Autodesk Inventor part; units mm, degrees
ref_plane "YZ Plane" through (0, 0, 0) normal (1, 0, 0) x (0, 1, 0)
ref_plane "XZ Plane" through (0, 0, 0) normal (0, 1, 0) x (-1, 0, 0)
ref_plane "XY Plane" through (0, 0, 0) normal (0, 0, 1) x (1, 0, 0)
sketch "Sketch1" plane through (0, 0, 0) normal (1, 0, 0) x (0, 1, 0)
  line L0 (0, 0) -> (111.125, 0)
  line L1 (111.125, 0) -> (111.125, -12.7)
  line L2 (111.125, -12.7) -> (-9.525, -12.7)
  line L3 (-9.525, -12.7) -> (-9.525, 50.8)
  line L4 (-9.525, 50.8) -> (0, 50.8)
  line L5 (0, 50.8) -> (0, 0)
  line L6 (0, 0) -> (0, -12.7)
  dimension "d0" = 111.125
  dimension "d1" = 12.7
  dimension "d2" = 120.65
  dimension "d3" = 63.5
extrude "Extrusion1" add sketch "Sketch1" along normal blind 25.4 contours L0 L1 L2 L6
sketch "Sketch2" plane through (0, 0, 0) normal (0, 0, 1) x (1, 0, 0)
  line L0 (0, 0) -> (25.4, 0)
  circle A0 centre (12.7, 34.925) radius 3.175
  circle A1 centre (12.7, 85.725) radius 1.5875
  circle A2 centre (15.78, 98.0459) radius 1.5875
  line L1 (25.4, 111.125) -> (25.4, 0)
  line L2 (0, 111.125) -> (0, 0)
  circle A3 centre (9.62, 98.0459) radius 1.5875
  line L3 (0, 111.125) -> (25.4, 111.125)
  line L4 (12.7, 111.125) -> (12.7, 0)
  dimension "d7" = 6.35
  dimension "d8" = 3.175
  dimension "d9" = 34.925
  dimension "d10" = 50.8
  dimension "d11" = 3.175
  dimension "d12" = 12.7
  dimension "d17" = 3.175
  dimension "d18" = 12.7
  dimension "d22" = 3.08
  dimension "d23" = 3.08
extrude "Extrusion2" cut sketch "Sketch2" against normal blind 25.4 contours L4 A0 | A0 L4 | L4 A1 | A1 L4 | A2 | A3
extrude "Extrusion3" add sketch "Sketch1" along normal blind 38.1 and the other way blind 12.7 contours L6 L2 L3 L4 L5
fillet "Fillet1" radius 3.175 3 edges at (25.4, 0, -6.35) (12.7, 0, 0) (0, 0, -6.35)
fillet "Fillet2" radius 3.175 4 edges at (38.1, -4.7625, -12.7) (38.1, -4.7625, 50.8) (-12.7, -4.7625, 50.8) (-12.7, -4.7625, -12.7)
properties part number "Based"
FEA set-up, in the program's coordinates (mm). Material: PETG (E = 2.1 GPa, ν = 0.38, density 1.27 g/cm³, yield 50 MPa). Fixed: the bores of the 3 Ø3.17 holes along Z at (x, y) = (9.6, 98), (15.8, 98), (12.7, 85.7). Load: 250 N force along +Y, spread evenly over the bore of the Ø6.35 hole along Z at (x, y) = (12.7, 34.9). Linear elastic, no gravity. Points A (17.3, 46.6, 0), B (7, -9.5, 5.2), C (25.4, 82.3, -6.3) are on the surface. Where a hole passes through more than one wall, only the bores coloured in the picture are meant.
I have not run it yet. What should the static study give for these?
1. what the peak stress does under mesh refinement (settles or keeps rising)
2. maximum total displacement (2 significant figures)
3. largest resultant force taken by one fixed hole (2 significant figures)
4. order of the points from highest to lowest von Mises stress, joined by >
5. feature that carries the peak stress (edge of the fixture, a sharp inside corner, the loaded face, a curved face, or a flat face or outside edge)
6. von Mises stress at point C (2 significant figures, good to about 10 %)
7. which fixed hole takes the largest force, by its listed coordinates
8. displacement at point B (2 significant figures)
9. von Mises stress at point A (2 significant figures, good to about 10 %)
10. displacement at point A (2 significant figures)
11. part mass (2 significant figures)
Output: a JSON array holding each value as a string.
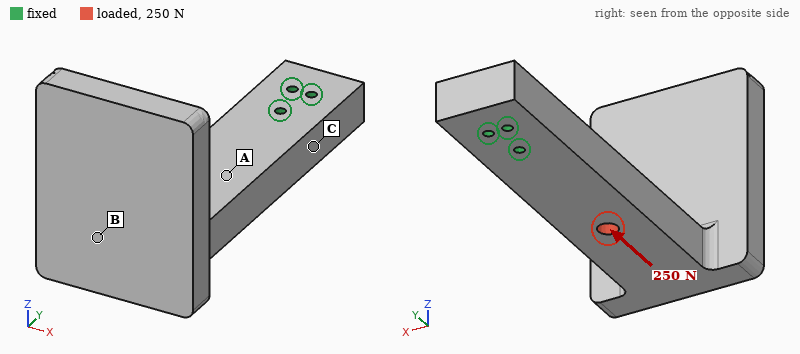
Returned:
["keeps rising", "25 µm", "160 N", "A > C > B", "edge of the fixture", "0.48 MPa", "(12.7, 85.7)", "22 µm", "0.88 MPa", "17 µm", "84 g"]
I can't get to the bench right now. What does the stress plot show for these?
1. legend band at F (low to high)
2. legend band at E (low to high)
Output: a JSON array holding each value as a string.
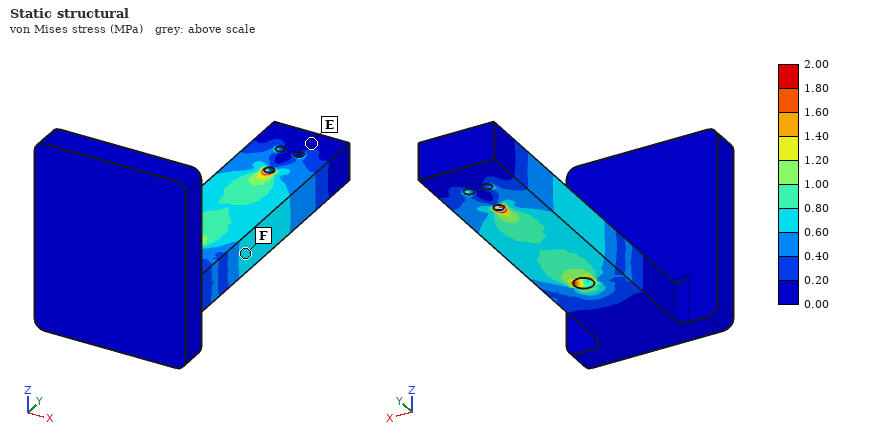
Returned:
["0.60 to 0.80 MPa", "0.00 to 0.20 MPa"]
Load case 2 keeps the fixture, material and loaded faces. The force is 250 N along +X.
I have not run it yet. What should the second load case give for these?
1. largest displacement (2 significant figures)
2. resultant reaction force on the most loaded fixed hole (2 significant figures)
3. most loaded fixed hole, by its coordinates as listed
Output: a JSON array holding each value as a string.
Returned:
["1.3 mm", "840 N", "(12.7, 85.7)"]
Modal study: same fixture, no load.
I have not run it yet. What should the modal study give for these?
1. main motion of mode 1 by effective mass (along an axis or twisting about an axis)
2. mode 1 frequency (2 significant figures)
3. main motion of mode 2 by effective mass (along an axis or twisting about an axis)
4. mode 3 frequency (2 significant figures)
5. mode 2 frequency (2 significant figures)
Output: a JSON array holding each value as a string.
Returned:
["along Z", "120 Hz", "along X", "380 Hz", "180 Hz"]
